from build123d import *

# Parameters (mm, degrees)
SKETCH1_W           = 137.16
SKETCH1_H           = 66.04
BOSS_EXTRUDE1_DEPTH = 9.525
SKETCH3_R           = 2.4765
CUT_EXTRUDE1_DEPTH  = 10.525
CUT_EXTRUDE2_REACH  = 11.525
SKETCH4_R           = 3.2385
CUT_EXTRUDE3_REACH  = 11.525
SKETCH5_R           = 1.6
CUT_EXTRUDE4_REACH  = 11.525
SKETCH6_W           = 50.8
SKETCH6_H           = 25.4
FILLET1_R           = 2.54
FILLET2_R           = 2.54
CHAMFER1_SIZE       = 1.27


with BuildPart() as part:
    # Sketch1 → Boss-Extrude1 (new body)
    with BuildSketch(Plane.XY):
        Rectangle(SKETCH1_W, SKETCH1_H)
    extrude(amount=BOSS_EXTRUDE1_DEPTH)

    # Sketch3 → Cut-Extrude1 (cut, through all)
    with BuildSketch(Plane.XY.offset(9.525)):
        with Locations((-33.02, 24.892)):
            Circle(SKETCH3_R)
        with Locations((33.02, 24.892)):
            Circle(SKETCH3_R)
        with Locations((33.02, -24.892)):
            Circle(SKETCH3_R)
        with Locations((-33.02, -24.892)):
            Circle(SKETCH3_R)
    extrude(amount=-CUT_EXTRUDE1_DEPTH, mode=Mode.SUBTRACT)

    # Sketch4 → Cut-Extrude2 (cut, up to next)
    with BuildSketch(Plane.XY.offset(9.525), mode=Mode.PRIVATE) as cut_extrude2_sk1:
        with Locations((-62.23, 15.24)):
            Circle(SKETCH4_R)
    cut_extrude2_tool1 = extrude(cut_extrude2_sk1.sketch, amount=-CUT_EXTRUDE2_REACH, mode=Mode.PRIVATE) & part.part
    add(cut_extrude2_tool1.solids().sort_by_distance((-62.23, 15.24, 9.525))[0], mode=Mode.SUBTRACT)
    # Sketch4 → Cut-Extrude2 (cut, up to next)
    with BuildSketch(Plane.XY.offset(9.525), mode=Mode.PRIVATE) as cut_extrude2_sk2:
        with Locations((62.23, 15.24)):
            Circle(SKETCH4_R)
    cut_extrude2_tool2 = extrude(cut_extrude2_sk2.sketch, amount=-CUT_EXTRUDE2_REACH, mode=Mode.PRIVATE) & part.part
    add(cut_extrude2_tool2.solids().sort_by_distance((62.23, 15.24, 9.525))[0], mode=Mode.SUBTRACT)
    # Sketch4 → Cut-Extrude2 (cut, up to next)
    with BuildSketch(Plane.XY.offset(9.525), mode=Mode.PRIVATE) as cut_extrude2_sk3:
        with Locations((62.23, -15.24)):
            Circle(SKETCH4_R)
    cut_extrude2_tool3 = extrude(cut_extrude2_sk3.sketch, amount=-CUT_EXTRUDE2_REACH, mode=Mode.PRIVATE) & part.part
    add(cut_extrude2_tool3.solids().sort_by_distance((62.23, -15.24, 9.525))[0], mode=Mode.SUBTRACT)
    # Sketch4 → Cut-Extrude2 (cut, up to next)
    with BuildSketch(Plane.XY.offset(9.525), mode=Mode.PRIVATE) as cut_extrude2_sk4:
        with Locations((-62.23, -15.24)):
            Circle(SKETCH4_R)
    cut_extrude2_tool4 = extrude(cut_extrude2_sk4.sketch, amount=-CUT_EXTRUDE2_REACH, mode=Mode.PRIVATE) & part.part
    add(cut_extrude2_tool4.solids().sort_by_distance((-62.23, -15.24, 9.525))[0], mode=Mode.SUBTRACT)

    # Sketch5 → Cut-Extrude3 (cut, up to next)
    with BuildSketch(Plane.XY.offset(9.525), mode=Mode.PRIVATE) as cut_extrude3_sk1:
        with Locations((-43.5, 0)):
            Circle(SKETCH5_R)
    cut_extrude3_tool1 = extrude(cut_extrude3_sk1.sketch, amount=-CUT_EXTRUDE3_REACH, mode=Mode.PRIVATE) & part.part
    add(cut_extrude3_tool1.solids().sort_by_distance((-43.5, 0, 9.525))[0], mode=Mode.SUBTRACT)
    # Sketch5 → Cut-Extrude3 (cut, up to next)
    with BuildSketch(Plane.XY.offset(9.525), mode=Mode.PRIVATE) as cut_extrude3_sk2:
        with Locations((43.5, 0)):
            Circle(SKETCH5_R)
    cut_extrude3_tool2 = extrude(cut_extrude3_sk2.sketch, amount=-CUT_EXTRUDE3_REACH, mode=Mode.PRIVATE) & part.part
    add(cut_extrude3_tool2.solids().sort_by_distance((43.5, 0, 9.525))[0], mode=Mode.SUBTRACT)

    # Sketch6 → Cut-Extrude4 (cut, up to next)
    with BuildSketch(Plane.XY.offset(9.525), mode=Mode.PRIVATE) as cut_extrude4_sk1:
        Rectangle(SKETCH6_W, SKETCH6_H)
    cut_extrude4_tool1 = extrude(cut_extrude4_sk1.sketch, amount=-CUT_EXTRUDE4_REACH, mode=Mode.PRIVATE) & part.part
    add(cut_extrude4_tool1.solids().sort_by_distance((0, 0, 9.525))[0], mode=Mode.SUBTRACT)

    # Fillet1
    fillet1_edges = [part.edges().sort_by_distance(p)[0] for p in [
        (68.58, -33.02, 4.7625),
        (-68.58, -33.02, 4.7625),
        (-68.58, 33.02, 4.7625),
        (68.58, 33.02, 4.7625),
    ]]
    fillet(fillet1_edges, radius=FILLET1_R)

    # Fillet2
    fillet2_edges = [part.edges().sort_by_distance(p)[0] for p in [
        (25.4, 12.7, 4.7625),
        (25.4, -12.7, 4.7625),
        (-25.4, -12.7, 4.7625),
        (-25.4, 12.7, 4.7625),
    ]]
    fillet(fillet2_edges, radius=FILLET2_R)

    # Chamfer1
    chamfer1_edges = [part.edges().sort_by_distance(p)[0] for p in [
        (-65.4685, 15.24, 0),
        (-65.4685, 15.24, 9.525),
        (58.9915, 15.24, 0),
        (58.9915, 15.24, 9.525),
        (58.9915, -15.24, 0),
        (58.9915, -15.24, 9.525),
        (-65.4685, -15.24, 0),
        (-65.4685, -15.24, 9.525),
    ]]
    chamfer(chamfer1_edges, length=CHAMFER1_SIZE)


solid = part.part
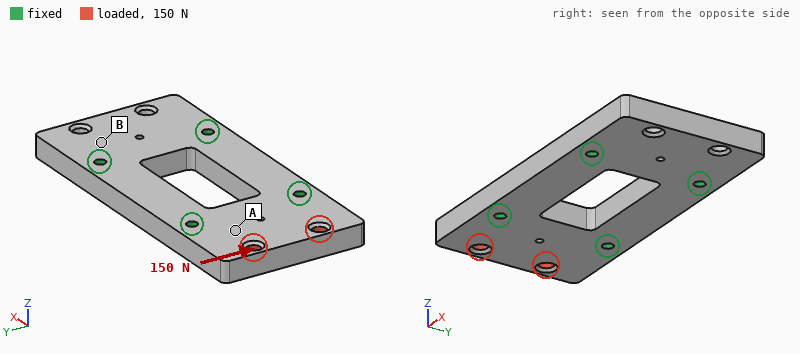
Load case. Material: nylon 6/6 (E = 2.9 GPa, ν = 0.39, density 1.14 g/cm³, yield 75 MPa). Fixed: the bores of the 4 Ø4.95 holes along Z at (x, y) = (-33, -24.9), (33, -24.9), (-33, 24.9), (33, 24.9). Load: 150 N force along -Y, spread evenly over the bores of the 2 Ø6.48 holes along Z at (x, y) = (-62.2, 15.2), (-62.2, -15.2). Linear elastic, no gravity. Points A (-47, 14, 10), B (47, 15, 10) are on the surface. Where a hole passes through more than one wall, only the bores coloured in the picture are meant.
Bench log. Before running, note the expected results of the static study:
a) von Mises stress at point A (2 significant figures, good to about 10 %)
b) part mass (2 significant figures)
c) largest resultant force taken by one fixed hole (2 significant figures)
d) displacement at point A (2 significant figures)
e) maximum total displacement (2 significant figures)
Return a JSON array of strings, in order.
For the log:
["0.58 MPa", "82 g", "110 N", "5.0 µm", "14 µm"]
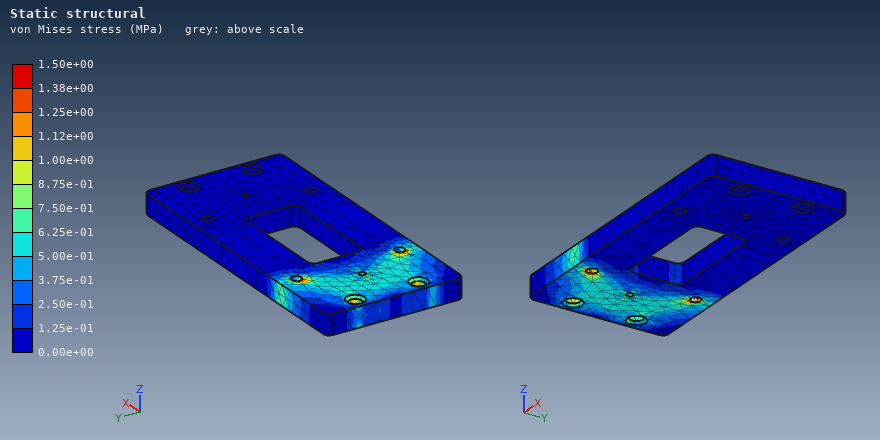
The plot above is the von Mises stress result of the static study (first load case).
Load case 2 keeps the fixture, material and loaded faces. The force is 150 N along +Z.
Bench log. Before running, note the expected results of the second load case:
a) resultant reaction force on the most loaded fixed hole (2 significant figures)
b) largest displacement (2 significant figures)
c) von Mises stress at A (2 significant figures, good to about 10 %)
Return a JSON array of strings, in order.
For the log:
["81 N", "0.20 mm", "2.2 MPa"]
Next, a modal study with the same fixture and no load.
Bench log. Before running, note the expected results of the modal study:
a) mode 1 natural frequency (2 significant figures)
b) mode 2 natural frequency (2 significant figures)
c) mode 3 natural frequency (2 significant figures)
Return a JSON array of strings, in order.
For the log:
["1500 Hz", "1600 Hz", "2700 Hz"]
